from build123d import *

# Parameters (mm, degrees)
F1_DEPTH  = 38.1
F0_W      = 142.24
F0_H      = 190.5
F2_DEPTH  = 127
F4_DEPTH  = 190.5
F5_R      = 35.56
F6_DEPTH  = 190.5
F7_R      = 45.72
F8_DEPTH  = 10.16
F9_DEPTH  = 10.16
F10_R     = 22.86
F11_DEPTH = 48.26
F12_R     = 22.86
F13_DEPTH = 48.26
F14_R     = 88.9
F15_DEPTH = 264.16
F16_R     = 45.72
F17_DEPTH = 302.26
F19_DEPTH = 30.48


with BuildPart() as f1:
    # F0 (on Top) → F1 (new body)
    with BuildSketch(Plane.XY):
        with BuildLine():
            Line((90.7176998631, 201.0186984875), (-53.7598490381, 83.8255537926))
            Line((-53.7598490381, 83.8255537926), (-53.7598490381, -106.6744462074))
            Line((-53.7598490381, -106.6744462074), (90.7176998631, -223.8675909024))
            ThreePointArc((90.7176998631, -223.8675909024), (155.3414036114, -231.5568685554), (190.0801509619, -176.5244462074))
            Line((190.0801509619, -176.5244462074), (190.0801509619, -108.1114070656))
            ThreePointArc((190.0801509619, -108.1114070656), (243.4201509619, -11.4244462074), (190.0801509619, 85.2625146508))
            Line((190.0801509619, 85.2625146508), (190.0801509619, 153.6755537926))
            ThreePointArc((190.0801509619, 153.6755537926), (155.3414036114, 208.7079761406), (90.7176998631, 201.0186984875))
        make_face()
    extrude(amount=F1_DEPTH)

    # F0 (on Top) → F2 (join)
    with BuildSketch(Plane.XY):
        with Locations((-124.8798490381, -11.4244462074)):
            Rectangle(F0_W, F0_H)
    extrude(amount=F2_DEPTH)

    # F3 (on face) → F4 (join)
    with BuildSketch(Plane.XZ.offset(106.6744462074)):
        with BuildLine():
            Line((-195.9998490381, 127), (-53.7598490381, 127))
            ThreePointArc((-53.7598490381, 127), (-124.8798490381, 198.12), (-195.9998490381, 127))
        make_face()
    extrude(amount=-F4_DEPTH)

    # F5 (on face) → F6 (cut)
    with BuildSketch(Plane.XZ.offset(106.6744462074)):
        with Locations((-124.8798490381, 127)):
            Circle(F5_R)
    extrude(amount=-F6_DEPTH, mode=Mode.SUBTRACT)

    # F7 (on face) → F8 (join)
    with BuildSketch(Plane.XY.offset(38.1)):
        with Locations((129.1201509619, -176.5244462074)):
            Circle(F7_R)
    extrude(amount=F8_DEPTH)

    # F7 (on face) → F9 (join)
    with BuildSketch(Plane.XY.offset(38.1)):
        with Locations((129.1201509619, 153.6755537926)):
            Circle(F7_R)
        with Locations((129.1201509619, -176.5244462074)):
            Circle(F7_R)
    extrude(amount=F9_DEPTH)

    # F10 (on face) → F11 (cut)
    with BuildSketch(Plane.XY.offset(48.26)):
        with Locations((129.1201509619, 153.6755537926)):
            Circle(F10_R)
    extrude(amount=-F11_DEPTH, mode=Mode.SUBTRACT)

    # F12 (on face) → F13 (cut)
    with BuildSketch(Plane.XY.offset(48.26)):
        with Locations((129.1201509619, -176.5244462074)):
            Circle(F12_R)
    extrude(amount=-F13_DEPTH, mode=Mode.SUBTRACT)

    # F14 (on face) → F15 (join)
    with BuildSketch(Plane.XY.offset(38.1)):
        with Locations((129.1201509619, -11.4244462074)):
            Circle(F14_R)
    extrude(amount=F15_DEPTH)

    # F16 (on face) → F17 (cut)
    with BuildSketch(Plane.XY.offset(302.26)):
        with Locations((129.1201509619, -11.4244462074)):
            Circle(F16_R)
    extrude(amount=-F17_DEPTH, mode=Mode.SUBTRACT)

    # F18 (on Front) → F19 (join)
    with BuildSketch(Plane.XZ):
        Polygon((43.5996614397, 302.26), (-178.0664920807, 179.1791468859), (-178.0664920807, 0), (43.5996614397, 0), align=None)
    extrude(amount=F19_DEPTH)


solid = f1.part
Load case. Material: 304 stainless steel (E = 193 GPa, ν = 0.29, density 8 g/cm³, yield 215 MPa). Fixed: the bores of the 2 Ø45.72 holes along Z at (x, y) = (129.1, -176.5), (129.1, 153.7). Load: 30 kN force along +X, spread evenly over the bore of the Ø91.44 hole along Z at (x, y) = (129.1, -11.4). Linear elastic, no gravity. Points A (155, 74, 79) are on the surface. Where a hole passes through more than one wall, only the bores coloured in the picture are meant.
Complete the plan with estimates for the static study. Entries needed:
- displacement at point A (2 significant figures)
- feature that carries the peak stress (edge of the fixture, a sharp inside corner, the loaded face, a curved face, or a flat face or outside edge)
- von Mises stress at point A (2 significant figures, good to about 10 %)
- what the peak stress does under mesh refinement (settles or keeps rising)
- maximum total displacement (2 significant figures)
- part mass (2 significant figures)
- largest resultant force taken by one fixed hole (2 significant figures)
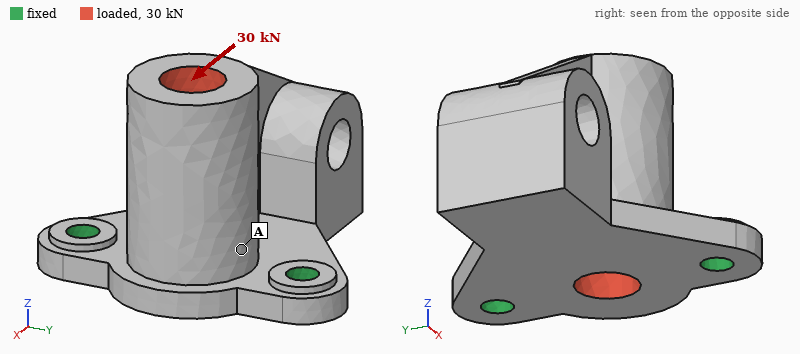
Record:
0.039 mm
edge of the fixture
5.4 MPa
keeps rising
0.19 mm
110 kg
16 kN
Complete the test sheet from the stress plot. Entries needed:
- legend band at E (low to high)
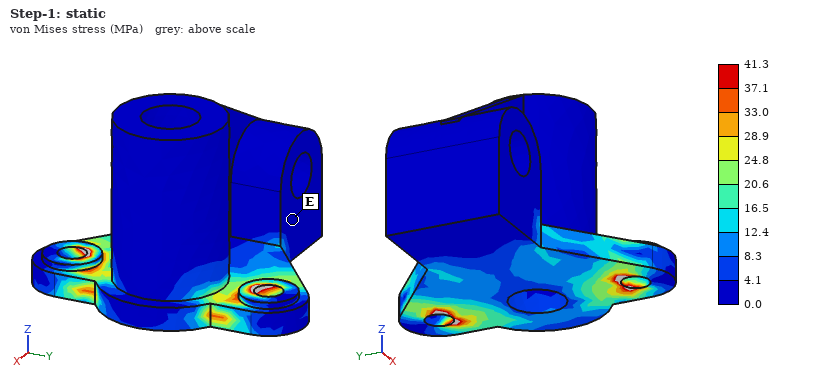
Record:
0.0 to 4.1 MPa
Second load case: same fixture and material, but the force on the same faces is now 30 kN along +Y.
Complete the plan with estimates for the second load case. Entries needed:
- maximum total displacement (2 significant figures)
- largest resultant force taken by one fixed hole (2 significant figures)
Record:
37 µm
22 kN
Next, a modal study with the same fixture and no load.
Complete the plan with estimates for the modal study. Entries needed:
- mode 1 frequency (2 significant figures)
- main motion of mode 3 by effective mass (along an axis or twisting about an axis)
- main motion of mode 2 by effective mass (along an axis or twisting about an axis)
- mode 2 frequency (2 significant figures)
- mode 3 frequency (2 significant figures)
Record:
210 Hz
along Z
along Y
620 Hz
940 Hz
